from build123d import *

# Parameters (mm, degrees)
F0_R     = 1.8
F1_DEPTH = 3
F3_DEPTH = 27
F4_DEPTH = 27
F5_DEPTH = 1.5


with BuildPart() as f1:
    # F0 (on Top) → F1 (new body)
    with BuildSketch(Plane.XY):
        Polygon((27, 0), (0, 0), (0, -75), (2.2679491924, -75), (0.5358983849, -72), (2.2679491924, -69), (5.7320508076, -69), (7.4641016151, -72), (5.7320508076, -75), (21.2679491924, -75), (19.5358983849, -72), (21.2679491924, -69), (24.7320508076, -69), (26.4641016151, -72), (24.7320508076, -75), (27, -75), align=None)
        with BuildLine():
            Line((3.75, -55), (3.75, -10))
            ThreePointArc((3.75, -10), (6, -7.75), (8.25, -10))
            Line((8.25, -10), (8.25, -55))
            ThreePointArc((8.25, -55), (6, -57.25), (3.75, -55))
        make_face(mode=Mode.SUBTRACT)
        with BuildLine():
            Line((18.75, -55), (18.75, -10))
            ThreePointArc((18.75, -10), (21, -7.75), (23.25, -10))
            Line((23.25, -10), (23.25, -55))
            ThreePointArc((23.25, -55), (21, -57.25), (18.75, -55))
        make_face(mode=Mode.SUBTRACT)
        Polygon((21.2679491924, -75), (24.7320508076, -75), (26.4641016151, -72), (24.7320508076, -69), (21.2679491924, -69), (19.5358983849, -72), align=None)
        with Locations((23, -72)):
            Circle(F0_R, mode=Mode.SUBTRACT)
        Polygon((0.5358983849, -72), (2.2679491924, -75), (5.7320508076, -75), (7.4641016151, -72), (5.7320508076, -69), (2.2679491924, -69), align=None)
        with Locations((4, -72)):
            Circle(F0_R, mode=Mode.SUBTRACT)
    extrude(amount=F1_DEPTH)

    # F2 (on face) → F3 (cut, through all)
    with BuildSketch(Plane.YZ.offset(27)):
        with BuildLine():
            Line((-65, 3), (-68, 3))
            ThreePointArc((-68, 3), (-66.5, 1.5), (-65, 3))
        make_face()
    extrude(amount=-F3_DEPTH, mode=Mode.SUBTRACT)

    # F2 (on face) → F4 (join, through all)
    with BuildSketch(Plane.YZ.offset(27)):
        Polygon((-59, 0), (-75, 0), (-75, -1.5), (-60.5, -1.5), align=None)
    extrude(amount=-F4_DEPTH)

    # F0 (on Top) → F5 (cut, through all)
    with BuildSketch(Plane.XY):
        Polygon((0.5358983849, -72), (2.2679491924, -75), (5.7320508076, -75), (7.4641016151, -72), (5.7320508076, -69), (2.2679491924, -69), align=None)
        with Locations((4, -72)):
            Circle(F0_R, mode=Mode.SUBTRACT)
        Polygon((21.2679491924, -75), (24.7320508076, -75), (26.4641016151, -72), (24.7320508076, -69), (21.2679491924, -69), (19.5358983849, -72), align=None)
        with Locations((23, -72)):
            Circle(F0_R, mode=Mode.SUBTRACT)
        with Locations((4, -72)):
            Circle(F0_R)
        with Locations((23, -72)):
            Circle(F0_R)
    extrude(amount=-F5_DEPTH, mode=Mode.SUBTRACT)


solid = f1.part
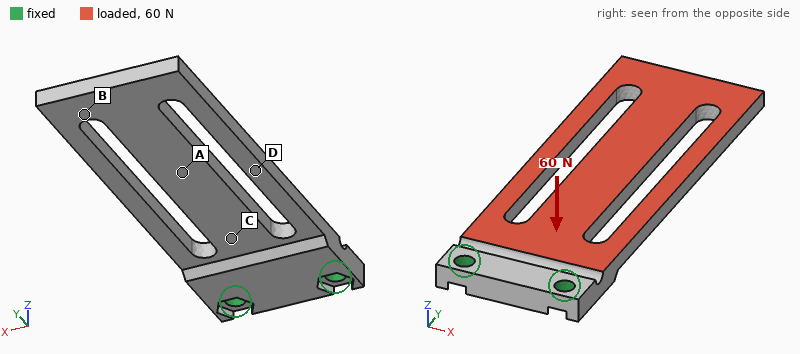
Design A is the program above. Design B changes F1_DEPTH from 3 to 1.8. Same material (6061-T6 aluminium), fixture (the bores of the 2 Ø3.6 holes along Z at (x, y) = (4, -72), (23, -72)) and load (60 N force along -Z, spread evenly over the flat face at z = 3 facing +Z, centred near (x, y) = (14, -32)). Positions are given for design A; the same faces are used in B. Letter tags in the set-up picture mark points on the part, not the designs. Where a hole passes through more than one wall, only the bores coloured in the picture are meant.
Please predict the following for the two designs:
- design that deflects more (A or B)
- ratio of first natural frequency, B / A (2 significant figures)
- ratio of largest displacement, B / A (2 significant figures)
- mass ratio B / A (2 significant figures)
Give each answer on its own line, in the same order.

B
0.67
3.7
0.65
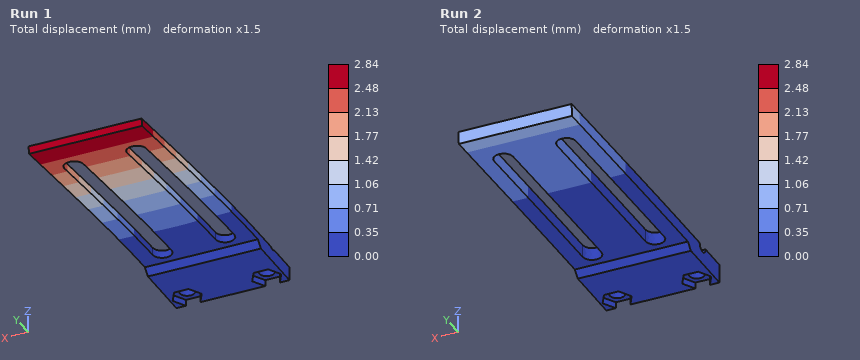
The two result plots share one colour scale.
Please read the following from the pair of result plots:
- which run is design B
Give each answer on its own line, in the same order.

Run 1
